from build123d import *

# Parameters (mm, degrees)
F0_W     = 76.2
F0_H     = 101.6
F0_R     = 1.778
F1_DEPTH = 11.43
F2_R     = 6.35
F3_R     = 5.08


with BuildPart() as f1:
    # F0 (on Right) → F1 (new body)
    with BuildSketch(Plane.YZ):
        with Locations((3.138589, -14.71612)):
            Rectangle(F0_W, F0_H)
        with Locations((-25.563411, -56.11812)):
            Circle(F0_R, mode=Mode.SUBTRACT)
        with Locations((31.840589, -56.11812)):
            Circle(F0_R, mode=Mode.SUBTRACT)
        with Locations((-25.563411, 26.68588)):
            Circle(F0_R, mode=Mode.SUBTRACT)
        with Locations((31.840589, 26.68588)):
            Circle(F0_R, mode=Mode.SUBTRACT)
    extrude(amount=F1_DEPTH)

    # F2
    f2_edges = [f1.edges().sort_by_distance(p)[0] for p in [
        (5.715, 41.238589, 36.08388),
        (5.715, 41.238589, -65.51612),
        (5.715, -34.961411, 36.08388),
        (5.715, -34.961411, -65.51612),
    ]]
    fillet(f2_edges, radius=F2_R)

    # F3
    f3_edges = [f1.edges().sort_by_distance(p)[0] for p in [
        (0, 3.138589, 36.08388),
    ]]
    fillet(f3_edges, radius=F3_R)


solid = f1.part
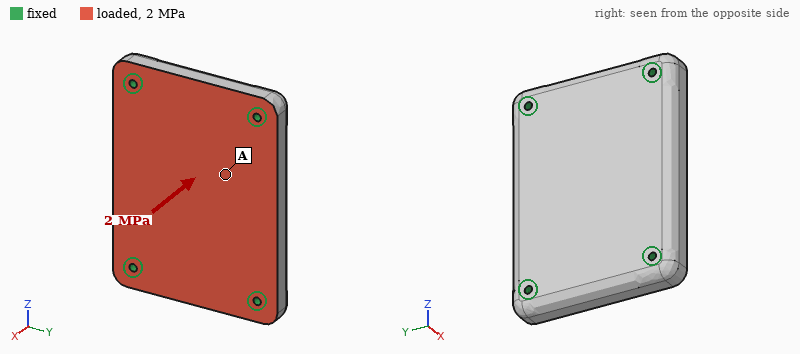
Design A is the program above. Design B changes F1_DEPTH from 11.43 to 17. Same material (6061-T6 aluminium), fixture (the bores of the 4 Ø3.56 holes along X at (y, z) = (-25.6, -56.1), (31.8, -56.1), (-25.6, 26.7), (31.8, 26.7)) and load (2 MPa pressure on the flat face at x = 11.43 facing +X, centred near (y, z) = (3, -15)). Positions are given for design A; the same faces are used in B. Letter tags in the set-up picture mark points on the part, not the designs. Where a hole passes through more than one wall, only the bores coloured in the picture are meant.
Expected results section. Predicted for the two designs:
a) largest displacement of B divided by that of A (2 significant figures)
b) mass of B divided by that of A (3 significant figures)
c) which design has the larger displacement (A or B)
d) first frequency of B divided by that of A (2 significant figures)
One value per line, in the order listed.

0.38
1.50
A
1.3
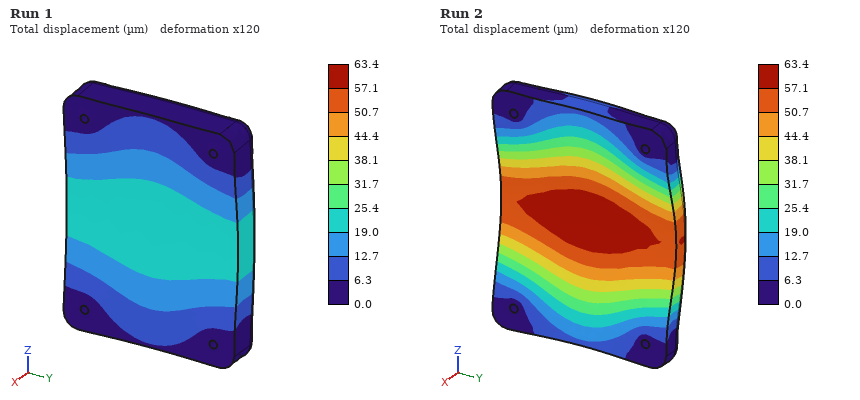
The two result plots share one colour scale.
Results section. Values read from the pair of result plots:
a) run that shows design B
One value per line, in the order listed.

Run 1
